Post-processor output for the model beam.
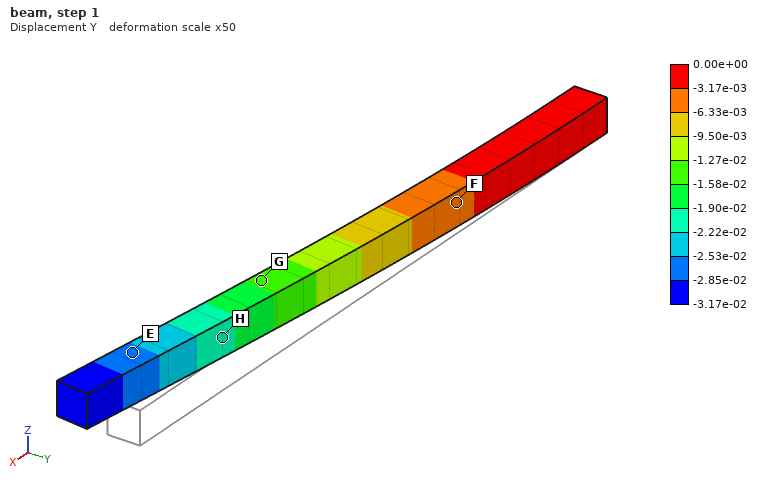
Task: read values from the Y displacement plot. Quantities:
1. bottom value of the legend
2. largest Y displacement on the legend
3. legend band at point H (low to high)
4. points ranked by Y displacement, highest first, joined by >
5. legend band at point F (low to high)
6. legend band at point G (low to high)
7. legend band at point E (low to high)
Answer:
-3.17e-02
0.00e+00
-2.22e-02 to -1.90e-02
F > G > H > E
-6.33e-03 to -3.17e-03
-1.58e-02 to -1.27e-02
-2.85e-02 to -2.53e-02
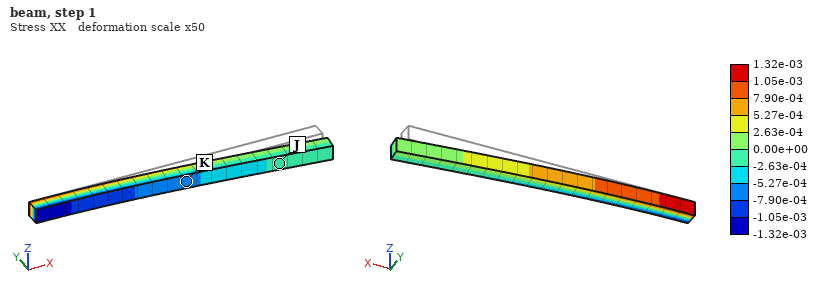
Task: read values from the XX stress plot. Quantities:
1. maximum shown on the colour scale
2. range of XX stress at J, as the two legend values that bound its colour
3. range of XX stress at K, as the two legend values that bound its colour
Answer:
1.32e-03
-2.63e-04 to 0.00e+00
-7.90e-04 to -5.27e-04
